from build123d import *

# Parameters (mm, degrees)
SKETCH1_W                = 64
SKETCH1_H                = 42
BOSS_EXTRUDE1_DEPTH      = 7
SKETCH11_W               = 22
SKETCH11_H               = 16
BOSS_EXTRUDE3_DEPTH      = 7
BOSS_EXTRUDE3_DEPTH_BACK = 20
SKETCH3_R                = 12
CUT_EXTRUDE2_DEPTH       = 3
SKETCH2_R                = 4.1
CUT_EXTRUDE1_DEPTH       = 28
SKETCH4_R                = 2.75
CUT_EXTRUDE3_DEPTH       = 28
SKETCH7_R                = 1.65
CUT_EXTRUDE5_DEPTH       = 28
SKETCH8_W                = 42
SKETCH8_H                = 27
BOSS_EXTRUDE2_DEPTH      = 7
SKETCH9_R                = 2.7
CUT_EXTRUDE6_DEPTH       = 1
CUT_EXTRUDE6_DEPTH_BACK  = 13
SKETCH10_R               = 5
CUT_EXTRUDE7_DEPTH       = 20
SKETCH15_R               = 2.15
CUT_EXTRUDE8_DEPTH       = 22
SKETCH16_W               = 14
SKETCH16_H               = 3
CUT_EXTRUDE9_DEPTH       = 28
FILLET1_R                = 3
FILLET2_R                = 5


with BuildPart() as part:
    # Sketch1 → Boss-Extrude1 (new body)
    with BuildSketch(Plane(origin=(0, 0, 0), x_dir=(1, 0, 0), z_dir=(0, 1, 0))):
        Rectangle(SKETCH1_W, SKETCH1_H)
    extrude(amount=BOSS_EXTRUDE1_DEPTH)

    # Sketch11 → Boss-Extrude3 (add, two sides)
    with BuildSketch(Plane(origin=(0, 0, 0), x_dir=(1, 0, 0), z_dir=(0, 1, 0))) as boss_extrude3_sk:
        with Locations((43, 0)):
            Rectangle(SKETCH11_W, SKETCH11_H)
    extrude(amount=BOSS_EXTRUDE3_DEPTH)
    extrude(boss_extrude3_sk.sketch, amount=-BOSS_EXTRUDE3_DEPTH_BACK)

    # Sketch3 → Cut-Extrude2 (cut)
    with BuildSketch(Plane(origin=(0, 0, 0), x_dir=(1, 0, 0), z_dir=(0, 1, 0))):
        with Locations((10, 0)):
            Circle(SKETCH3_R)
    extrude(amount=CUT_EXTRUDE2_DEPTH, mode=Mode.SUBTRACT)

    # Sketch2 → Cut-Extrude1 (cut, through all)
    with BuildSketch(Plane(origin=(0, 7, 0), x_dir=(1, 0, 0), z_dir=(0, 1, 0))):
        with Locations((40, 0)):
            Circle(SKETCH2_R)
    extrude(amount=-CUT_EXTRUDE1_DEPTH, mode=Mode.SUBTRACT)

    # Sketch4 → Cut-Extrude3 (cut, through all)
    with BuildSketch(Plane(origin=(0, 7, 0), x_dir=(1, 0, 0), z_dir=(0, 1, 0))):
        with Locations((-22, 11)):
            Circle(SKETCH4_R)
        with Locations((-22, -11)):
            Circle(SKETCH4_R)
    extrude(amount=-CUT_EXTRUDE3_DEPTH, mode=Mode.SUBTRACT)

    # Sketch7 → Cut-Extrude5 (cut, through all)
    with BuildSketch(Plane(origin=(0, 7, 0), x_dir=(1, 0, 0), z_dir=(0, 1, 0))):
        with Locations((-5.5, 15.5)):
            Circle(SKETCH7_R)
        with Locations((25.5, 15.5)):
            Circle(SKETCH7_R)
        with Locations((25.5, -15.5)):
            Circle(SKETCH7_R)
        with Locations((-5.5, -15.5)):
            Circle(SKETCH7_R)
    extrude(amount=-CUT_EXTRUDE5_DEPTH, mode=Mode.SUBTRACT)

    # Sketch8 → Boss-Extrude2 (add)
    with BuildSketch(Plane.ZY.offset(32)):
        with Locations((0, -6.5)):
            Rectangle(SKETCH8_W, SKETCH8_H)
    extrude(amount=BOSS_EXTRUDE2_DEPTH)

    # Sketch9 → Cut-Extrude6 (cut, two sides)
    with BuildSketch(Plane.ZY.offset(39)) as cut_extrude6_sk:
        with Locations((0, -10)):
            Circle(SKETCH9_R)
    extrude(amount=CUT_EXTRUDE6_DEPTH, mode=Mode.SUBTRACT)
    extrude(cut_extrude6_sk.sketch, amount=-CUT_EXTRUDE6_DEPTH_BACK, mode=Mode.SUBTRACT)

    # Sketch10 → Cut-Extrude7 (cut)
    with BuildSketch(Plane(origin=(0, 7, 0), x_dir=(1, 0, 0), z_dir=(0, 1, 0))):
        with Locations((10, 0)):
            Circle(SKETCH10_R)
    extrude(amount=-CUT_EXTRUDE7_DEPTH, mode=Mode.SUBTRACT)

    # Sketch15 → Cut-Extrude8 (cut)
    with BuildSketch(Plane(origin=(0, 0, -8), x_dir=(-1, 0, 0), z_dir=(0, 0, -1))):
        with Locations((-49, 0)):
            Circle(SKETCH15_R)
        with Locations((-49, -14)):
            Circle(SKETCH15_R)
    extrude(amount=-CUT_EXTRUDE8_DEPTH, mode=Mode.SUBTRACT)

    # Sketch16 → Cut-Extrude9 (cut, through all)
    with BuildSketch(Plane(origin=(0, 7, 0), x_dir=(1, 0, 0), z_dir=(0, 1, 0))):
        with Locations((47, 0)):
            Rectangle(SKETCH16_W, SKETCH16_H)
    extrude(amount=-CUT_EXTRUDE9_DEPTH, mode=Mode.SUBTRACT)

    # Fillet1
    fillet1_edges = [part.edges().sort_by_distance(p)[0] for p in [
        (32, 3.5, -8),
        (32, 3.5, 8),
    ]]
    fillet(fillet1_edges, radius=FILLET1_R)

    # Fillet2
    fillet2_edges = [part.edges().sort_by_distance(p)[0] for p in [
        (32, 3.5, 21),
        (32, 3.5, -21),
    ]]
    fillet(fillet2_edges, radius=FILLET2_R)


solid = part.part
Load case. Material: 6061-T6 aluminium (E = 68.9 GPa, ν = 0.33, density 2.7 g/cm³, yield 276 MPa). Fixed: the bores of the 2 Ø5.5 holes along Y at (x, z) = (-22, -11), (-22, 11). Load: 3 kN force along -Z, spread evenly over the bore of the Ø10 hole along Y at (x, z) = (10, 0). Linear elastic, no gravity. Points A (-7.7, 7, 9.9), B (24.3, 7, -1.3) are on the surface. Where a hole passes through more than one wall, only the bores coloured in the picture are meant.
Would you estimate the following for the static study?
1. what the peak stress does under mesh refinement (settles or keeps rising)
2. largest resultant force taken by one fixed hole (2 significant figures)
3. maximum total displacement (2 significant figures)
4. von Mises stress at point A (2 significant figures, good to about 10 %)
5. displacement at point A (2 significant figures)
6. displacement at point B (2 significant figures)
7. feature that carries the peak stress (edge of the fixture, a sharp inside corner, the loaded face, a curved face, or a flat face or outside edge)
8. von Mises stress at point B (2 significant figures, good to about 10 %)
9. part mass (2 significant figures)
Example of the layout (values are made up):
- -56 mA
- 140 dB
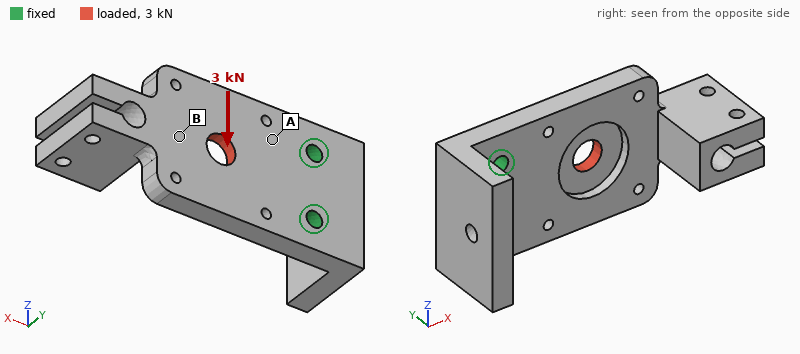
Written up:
- keeps rising
- 4.0 kN
- 68 µm
- 29 MPa
- 13 µm
- 49 µm
- edge of the fixture
- 12 MPa
- 84 g
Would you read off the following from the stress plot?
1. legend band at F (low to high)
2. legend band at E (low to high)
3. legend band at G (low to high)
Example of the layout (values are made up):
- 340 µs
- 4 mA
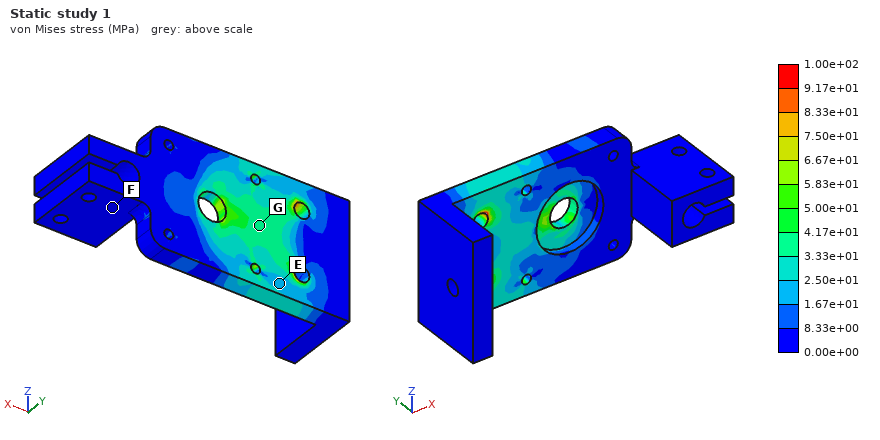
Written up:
- 0.00e+00 to 8.33e+00 MPa
- 1.67e+01 to 2.50e+01 MPa
- 3.33e+01 to 4.17e+01 MPa
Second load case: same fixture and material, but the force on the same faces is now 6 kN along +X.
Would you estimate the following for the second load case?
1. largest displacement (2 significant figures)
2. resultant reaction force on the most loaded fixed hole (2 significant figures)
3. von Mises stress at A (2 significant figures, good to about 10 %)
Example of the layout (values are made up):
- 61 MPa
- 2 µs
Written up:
- 0.21 mm
- 3.0 kN
- 51 MPa
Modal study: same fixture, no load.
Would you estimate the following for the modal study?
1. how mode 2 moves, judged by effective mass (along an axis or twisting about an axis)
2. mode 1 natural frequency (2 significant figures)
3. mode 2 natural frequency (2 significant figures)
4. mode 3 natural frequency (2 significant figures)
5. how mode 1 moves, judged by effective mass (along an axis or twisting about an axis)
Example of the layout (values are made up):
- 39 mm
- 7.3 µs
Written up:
- along Z
- 850 Hz
- 2500 Hz
- 3800 Hz
- along Y
